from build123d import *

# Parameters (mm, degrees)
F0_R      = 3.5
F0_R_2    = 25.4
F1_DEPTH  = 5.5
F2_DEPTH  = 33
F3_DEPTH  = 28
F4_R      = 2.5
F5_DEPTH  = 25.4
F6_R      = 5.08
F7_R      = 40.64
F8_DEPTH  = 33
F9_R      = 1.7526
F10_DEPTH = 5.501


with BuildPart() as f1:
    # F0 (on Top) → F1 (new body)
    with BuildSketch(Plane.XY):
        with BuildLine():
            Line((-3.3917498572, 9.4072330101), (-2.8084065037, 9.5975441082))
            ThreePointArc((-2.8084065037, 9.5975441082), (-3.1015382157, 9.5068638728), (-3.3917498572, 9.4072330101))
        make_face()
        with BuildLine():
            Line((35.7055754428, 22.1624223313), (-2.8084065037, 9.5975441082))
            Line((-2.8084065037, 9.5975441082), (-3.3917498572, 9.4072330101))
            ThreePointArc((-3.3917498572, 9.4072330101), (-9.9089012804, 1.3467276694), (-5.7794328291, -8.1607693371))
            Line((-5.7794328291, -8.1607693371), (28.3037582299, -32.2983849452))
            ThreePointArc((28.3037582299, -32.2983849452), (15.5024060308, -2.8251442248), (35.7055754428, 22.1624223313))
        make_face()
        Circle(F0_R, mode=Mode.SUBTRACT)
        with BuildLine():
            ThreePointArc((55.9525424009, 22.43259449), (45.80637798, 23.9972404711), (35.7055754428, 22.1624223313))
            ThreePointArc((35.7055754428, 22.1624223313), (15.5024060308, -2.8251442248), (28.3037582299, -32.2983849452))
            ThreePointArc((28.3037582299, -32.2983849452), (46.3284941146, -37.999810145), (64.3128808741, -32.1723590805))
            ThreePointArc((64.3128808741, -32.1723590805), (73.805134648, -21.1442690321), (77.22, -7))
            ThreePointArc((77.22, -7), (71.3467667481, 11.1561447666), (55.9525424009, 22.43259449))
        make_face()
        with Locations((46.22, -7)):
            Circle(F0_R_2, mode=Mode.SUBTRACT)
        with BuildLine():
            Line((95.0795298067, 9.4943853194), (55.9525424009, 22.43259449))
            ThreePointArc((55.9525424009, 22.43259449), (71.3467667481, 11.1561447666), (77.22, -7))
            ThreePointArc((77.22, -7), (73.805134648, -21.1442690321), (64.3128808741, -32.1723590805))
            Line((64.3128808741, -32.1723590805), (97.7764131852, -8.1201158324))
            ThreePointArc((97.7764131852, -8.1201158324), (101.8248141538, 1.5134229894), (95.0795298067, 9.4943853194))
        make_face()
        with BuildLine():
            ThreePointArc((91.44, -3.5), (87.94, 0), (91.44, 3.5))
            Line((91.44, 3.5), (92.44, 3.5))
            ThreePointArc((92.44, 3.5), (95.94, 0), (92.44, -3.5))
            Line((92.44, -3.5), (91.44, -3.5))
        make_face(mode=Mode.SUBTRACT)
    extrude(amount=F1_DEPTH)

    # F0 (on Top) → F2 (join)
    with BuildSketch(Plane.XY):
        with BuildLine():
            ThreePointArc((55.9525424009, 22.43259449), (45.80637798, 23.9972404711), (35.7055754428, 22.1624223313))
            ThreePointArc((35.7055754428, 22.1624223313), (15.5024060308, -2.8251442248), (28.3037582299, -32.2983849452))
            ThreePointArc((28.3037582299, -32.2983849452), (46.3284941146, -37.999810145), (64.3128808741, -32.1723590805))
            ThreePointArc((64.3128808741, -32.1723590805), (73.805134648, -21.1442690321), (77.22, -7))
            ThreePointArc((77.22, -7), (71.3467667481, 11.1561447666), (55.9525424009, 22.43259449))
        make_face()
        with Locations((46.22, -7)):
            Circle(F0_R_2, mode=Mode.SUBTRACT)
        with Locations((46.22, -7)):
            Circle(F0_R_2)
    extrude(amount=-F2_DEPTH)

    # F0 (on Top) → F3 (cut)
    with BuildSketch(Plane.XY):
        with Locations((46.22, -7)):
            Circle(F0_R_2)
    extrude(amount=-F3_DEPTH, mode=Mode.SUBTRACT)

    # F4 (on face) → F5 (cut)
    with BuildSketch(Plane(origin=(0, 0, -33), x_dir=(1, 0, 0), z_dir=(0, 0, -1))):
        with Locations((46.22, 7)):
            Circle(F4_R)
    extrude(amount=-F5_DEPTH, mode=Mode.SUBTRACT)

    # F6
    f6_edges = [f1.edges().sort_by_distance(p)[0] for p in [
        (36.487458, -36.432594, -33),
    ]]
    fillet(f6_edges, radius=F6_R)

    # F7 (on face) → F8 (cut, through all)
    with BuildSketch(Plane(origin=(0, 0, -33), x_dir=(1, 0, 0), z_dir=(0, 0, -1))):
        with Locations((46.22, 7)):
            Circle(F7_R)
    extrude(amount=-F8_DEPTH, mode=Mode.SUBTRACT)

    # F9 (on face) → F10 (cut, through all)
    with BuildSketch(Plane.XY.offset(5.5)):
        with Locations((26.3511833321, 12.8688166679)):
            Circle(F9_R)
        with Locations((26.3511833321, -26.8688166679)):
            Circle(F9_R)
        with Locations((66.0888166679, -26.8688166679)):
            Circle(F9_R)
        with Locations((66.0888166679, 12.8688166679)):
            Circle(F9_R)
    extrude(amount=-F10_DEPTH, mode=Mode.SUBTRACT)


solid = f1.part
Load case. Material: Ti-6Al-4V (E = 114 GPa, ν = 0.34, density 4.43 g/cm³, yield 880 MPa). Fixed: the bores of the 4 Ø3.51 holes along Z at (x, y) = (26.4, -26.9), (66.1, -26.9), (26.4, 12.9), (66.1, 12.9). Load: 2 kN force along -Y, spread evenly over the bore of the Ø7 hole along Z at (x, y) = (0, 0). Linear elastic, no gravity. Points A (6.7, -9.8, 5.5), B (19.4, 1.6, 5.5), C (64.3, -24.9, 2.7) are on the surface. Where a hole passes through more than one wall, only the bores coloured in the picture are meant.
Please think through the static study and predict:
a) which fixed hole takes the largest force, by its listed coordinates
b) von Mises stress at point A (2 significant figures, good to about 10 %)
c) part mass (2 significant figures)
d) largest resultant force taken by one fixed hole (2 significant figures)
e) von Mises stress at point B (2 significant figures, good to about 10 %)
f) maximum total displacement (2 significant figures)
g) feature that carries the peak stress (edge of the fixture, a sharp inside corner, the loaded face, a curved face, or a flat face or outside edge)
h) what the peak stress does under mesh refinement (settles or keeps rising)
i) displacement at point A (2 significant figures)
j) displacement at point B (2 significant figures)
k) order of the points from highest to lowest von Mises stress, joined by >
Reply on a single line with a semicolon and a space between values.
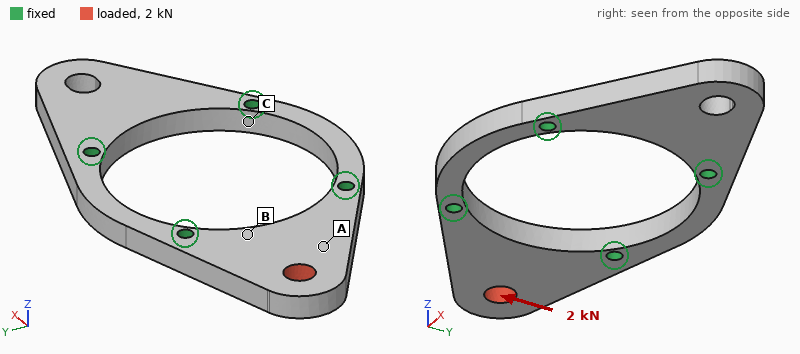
(26.4, -26.9); 22 MPa; 58 g; 1.7 kN; 12 MPa; 16 µm; edge of the fixture; keeps rising; 7.9 µm; 3.2 µm; A > B > C
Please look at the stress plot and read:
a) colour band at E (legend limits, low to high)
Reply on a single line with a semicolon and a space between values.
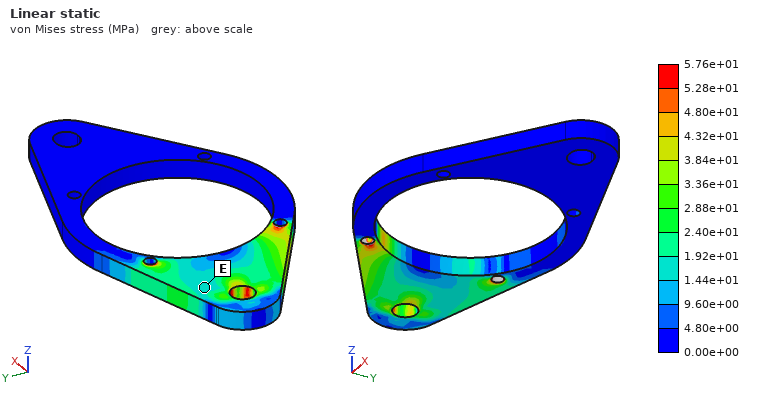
1.44e+01 to 1.92e+01 MPa
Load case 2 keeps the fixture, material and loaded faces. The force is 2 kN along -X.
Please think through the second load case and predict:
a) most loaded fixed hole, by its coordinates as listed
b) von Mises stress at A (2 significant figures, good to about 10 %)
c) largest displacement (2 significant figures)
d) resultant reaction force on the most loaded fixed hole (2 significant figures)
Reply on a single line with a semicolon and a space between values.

(26.4, 12.9); 13 MPa; 7.0 µm; 1.4 kN
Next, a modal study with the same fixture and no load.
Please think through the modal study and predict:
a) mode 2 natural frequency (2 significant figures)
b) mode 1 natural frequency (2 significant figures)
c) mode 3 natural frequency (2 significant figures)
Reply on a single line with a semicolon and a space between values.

3500 Hz; 3400 Hz; 12 kHz
